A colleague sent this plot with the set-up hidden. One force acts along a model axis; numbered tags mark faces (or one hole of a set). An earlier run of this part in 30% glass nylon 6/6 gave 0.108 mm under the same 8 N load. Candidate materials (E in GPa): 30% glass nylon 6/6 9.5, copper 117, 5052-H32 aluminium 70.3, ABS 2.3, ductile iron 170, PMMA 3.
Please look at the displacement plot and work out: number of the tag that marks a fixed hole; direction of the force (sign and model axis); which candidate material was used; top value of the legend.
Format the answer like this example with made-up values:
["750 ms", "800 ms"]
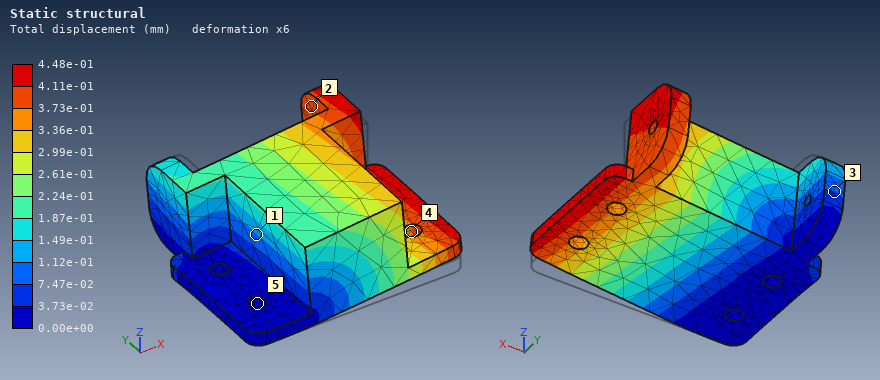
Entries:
["5", "+Z", "ABS", "4.48e-01 mm"]
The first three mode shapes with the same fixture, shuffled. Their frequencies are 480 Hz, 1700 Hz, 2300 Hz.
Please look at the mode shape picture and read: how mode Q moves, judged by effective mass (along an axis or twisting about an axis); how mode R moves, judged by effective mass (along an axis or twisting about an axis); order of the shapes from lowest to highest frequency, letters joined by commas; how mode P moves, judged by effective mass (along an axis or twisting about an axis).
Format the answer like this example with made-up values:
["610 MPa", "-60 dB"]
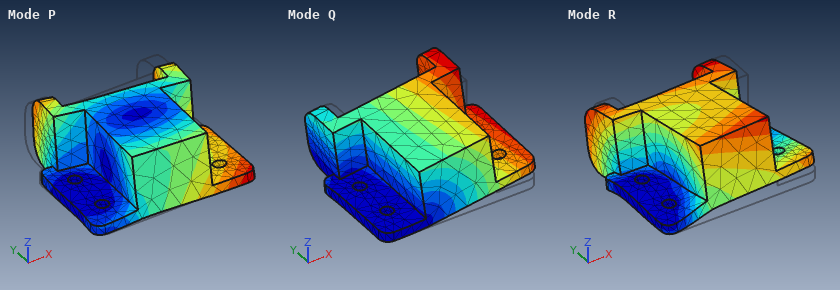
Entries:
["along Z", "along Y", "Q, R, P", "along Y"]
